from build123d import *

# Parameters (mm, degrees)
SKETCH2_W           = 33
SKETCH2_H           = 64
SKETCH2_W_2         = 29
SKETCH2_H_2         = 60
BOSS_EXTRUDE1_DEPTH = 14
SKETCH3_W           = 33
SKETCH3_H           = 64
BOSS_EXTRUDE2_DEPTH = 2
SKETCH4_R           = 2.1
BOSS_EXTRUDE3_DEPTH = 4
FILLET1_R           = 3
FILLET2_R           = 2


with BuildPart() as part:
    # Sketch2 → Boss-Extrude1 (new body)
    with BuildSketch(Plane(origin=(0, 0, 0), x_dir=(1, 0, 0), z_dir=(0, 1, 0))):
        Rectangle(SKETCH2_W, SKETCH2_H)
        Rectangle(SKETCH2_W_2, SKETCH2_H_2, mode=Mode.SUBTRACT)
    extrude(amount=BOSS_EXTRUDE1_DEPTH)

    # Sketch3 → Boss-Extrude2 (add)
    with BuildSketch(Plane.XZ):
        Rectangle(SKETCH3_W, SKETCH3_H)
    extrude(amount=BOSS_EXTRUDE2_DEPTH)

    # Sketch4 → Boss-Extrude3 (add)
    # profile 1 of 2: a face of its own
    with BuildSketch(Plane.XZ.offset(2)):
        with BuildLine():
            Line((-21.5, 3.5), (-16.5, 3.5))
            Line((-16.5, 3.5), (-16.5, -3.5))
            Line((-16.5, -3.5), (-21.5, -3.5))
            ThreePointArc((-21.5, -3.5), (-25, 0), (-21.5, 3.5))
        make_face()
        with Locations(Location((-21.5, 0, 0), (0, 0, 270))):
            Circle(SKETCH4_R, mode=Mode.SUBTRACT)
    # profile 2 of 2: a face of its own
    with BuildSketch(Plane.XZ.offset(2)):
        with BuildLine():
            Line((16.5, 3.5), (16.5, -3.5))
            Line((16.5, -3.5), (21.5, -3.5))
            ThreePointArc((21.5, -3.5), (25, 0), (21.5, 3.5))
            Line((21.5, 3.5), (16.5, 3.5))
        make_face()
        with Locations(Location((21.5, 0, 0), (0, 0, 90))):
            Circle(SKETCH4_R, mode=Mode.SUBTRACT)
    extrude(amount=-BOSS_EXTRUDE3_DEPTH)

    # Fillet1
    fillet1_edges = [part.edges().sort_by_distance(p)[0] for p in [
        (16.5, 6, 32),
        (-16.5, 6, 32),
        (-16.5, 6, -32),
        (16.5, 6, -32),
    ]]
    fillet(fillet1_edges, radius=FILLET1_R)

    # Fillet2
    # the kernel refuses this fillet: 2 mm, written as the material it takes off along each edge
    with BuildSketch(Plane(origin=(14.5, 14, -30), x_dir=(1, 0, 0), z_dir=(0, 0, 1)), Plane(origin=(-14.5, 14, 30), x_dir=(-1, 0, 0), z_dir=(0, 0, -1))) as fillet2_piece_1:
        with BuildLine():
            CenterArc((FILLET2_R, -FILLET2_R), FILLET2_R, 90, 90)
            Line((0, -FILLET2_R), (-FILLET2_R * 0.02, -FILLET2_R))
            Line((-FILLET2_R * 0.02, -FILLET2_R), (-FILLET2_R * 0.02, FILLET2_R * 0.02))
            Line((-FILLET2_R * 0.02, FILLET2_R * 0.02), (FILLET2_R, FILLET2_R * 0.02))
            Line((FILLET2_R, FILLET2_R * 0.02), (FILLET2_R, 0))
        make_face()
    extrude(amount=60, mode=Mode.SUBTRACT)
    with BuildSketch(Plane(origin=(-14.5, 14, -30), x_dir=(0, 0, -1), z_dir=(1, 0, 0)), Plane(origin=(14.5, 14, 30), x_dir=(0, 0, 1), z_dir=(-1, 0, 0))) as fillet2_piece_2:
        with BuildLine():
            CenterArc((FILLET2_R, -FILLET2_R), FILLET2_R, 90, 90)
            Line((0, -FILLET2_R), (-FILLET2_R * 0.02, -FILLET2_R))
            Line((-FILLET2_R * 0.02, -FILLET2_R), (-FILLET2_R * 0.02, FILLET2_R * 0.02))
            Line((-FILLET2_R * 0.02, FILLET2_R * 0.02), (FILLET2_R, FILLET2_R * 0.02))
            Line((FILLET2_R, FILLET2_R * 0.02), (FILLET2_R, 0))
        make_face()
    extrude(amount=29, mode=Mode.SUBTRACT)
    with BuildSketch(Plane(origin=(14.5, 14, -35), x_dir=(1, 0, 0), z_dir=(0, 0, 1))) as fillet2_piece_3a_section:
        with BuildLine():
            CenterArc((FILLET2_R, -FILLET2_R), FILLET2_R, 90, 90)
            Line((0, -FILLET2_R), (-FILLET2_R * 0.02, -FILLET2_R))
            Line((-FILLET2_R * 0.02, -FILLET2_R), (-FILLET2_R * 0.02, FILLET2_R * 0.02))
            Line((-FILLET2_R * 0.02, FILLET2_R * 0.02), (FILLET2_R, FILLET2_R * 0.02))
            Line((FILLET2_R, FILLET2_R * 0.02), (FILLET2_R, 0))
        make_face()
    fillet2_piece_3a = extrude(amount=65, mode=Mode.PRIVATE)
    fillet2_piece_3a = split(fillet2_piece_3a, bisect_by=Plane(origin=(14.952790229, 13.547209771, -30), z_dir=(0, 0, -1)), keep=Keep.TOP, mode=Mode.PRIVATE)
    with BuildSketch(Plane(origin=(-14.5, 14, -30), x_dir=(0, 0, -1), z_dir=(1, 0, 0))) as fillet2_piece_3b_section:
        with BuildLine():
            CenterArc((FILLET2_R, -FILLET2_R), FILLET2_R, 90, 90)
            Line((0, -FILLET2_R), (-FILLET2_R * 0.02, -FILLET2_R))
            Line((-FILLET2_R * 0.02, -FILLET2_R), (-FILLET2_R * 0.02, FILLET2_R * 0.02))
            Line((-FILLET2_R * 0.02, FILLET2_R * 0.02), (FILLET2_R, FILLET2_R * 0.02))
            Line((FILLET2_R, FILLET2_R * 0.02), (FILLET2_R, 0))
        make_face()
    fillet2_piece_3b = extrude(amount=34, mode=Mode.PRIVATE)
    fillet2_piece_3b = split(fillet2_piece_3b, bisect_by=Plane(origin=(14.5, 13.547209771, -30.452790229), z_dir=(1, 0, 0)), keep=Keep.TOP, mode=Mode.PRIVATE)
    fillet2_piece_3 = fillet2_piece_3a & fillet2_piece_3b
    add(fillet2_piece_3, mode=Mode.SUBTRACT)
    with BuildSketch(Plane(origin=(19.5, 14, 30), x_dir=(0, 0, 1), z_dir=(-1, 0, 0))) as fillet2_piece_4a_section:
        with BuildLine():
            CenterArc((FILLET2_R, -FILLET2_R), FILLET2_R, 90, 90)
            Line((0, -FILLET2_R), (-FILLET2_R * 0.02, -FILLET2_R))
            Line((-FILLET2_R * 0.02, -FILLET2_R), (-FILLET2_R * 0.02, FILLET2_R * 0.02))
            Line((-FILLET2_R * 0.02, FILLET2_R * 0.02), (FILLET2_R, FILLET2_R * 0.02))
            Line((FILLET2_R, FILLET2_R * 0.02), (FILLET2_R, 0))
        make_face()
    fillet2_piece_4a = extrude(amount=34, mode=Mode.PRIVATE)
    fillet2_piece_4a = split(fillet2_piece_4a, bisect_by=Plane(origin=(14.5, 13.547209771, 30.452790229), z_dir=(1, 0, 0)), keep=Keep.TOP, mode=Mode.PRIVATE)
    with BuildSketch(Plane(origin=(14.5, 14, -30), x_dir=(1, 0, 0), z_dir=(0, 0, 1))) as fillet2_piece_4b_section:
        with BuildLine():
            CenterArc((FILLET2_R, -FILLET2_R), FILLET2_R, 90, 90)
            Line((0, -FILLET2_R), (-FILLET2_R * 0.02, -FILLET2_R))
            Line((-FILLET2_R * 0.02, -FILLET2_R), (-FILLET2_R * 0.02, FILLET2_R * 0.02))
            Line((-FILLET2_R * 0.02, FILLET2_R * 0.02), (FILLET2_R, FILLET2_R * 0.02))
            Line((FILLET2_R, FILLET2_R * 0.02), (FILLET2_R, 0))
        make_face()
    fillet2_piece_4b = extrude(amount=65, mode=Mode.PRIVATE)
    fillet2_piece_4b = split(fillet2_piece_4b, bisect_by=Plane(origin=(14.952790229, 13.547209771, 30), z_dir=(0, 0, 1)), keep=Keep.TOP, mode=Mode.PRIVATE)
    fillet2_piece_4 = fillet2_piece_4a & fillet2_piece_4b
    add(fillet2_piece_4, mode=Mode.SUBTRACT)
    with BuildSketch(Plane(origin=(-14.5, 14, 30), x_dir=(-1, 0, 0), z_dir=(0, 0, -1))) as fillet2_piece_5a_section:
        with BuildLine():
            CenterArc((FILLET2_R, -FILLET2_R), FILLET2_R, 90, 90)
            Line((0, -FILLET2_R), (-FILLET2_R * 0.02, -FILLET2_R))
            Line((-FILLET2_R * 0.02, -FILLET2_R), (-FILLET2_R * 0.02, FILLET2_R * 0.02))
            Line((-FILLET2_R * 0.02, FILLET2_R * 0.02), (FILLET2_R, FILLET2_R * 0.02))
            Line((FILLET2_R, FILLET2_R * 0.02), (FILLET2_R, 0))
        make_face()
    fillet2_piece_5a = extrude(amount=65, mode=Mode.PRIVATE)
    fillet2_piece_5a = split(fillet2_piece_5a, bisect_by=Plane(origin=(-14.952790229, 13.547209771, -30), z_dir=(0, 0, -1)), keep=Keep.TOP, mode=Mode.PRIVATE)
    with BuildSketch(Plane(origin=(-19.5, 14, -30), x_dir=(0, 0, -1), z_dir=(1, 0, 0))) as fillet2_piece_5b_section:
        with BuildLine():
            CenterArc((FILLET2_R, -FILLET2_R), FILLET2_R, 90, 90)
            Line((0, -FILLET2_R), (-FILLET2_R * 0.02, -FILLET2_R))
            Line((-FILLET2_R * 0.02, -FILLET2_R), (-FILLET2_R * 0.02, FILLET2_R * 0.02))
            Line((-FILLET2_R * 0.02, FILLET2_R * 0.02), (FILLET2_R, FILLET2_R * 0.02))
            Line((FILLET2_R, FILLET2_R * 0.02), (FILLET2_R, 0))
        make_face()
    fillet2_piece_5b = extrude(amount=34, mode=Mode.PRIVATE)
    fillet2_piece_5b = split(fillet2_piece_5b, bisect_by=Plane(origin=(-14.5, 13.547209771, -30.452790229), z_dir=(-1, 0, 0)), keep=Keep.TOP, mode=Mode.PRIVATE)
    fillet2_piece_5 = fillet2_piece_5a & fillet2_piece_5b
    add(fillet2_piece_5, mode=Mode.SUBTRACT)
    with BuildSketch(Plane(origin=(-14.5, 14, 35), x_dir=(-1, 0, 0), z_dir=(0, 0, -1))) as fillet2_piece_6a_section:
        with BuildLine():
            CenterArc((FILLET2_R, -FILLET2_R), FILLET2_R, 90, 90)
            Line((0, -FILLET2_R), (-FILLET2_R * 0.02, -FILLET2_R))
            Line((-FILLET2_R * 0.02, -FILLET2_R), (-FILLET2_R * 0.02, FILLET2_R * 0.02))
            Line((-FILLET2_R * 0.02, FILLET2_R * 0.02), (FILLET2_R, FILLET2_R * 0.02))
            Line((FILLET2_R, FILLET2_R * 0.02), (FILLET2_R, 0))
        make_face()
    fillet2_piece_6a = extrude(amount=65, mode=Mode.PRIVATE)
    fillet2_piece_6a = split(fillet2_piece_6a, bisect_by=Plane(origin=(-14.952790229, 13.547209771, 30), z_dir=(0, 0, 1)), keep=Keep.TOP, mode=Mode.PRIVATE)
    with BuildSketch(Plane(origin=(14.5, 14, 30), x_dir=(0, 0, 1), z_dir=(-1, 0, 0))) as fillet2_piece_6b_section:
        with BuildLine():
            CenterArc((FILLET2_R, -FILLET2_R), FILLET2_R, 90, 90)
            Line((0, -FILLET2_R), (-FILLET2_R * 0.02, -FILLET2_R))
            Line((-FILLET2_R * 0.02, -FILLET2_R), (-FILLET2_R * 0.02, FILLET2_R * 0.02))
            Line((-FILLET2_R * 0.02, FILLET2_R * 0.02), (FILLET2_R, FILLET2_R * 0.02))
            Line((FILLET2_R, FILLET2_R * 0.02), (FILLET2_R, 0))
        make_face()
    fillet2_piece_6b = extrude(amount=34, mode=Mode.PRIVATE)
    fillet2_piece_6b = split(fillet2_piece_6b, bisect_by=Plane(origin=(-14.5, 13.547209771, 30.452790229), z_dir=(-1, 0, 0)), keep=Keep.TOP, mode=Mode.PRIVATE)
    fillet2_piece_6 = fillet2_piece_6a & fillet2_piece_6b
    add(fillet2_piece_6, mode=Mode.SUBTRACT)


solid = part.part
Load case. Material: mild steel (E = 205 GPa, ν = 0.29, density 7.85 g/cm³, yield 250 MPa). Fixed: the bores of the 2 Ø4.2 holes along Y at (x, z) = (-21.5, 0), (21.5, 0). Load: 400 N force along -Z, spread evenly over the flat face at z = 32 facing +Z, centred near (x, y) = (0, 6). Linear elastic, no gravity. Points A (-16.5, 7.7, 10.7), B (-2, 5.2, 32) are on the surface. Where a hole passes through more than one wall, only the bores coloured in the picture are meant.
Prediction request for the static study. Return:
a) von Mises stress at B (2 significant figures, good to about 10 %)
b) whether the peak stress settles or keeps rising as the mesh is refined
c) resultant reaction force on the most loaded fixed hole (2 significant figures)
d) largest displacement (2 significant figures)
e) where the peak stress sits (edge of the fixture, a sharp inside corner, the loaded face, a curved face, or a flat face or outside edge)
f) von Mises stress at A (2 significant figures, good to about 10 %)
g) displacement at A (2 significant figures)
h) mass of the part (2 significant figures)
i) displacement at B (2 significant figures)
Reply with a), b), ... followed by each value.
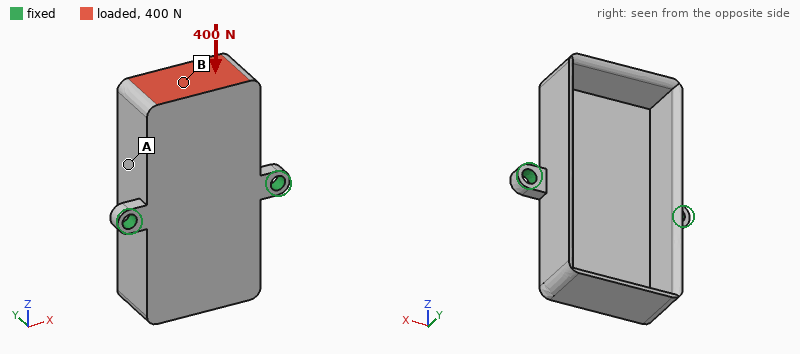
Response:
a) 22 MPa
b) keeps rising
c) 200 N
d) 41 µm
e) edge of the fixture
f) 8.6 MPa
g) 9.2 µm
h) 74 g
i) 28 µm
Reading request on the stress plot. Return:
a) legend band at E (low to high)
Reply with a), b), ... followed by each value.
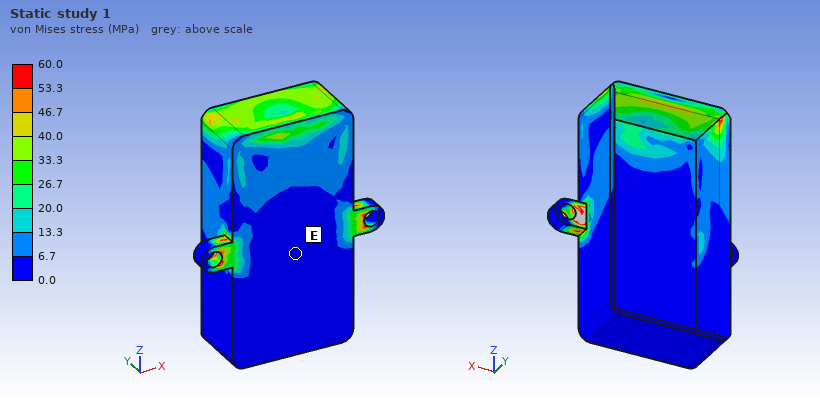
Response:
a) 0.0 to 6.7 MPa
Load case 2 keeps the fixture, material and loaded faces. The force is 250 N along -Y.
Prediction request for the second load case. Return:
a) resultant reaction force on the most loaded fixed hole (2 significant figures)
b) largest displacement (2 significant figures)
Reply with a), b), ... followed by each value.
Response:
a) 130 N
b) 88 µm
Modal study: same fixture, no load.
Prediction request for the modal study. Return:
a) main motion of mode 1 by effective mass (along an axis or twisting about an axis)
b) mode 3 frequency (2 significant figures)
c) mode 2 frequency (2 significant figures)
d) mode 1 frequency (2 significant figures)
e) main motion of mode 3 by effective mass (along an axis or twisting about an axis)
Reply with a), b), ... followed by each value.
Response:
a) twisting about X
b) 5700 Hz
c) 3000 Hz
d) 1600 Hz
e) along Y
